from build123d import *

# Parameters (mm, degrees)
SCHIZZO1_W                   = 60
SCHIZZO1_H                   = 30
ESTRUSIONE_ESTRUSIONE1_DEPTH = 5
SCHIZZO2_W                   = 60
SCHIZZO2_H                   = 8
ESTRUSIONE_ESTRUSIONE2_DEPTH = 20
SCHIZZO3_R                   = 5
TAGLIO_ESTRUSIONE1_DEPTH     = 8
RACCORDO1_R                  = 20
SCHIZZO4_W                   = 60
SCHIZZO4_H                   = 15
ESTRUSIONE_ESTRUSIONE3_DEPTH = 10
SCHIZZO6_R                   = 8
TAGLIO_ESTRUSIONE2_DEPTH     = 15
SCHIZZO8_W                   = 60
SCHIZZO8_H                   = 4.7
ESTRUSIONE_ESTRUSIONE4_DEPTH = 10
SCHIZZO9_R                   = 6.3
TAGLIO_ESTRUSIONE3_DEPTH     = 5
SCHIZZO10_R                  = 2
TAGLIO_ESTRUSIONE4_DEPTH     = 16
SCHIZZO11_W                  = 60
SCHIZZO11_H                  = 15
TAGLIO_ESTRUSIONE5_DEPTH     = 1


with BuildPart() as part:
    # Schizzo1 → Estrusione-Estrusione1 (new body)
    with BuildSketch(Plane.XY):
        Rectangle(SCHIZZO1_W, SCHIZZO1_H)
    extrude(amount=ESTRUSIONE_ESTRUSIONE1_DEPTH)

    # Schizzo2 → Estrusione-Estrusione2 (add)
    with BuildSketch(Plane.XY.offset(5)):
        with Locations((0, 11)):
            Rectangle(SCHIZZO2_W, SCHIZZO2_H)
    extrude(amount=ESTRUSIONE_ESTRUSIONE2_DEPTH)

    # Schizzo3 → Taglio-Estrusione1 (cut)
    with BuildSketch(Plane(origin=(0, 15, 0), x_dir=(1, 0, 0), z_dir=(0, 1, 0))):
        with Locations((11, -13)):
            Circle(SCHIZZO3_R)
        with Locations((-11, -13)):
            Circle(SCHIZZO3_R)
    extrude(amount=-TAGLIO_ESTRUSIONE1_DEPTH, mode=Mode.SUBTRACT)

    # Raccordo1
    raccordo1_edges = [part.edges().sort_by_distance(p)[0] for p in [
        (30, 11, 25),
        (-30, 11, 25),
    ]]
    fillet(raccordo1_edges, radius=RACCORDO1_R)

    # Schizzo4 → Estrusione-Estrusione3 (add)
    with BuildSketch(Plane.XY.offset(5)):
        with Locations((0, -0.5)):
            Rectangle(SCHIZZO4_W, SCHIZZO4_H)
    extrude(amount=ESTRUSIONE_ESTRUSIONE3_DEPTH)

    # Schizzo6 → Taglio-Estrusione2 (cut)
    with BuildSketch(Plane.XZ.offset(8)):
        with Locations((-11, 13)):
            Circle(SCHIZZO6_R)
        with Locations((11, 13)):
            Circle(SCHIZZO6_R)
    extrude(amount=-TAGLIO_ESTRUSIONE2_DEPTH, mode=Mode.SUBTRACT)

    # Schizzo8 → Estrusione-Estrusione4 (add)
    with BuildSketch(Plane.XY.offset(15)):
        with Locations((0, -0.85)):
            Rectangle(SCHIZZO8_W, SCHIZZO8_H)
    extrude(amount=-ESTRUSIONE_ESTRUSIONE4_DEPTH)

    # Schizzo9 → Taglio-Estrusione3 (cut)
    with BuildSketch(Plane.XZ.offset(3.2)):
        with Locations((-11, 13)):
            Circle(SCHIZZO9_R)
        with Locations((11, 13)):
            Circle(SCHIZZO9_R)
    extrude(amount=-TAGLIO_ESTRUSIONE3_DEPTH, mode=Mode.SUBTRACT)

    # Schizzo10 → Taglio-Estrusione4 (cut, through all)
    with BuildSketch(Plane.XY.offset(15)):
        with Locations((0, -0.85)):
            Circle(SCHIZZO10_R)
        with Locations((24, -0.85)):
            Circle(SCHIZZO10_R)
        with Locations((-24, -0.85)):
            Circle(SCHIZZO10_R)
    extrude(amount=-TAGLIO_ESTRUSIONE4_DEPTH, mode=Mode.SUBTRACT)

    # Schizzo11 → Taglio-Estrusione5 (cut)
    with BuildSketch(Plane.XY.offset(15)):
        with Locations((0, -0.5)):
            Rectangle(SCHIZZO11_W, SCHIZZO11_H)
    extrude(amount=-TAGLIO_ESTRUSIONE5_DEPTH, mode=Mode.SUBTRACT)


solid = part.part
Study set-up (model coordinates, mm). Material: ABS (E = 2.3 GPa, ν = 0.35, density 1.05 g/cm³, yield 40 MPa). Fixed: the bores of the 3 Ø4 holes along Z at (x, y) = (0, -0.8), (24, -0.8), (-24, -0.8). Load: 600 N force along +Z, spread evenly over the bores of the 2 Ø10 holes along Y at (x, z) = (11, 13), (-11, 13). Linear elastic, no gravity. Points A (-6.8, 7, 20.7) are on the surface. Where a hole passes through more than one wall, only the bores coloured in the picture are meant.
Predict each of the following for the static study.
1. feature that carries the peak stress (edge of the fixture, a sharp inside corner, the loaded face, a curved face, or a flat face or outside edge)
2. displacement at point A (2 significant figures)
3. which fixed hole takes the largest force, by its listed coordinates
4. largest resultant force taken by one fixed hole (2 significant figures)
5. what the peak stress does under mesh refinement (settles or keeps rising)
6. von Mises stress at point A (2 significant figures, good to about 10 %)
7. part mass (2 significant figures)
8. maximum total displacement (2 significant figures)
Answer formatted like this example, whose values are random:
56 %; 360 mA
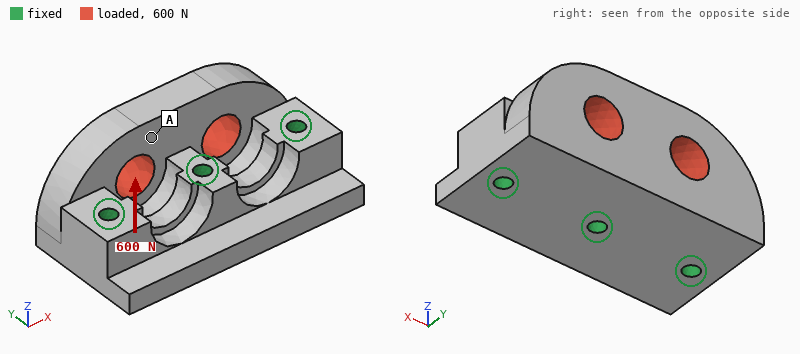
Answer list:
edge of the fixture; 56 µm; (0, -0.8); 280 N; keeps rising; 1.7 MPa; 21 g; 83 µm
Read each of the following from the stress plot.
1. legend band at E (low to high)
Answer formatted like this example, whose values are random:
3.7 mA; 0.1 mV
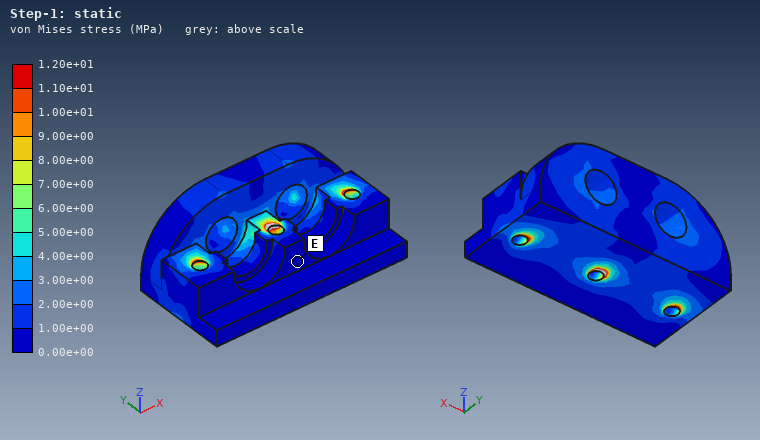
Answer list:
0.00e+00 to 1.00e+00 MPa
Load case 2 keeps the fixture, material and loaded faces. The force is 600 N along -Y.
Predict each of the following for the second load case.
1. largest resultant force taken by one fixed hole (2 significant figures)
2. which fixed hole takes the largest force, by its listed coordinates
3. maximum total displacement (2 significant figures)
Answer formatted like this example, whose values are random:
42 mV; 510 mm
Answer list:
350 N; (0, -0.8); 99 µm
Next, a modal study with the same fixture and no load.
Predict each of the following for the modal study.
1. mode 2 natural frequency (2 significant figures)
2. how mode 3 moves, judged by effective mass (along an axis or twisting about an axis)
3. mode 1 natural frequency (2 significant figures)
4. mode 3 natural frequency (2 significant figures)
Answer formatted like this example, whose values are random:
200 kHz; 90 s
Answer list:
6000 Hz; along Z; 4500 Hz; 7800 Hz
